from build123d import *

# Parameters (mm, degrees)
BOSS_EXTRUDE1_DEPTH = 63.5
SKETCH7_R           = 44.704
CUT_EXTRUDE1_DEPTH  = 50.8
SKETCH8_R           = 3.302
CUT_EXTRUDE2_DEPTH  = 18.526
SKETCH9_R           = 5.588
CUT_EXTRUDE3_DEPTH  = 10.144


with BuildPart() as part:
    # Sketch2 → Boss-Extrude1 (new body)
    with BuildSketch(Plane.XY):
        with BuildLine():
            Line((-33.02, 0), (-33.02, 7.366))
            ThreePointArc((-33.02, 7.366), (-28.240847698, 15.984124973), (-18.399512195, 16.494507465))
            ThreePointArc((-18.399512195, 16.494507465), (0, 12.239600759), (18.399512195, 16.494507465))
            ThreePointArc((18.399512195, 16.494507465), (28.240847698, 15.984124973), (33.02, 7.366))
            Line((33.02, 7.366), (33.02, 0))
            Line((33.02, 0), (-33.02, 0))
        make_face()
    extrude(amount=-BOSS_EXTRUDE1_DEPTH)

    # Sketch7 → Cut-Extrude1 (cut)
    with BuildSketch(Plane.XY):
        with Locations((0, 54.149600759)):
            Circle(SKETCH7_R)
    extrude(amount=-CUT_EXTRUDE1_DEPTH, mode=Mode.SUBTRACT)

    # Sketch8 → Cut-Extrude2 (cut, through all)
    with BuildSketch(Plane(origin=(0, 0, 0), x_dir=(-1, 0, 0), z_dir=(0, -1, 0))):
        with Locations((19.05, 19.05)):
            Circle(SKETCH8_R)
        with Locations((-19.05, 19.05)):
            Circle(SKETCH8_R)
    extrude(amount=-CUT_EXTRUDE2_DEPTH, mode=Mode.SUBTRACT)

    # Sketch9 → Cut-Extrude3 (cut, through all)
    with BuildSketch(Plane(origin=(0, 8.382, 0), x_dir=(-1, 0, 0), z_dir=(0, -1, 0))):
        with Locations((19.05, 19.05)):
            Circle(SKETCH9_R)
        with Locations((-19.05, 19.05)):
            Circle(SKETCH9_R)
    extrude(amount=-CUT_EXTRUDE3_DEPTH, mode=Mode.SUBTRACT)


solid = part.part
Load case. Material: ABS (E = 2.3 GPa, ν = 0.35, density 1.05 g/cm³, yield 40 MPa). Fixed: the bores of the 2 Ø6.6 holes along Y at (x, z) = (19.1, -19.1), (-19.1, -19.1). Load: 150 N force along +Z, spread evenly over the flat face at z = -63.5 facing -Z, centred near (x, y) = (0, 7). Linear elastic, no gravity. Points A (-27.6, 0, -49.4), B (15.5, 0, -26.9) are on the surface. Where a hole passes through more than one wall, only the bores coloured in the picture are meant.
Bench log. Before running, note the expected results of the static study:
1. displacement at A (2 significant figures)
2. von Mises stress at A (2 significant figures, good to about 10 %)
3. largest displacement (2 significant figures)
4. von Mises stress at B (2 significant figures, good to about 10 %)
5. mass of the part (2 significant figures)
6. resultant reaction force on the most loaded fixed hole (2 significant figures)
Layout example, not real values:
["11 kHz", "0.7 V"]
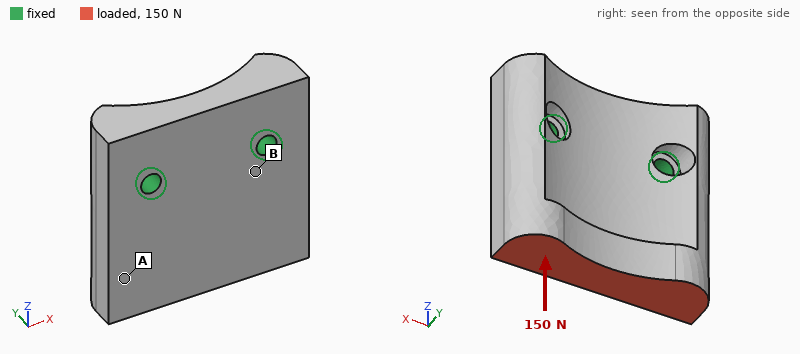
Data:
["10 µm", "0.11 MPa", "20 µm", "0.20 MPa", "56 g", "75 N"]
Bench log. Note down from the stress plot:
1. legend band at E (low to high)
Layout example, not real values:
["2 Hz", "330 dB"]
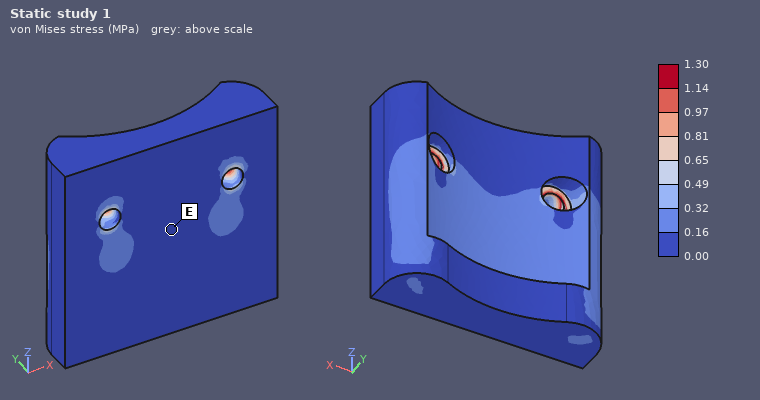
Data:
["0.00 to 0.16 MPa"]
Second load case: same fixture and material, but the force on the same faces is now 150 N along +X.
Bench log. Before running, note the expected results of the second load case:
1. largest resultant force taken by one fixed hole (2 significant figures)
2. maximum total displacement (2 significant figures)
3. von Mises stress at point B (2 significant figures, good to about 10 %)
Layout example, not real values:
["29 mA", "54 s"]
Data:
["180 N", "31 µm", "0.86 MPa"]
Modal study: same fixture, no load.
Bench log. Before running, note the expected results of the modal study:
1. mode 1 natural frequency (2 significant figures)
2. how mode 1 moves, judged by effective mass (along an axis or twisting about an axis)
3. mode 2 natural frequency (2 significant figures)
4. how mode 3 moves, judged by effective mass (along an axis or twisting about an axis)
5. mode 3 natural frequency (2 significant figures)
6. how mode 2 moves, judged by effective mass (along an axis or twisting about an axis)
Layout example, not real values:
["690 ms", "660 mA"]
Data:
["1000 Hz", "along Y", "1900 Hz", "along X", "2900 Hz", "twisting about Z"]
